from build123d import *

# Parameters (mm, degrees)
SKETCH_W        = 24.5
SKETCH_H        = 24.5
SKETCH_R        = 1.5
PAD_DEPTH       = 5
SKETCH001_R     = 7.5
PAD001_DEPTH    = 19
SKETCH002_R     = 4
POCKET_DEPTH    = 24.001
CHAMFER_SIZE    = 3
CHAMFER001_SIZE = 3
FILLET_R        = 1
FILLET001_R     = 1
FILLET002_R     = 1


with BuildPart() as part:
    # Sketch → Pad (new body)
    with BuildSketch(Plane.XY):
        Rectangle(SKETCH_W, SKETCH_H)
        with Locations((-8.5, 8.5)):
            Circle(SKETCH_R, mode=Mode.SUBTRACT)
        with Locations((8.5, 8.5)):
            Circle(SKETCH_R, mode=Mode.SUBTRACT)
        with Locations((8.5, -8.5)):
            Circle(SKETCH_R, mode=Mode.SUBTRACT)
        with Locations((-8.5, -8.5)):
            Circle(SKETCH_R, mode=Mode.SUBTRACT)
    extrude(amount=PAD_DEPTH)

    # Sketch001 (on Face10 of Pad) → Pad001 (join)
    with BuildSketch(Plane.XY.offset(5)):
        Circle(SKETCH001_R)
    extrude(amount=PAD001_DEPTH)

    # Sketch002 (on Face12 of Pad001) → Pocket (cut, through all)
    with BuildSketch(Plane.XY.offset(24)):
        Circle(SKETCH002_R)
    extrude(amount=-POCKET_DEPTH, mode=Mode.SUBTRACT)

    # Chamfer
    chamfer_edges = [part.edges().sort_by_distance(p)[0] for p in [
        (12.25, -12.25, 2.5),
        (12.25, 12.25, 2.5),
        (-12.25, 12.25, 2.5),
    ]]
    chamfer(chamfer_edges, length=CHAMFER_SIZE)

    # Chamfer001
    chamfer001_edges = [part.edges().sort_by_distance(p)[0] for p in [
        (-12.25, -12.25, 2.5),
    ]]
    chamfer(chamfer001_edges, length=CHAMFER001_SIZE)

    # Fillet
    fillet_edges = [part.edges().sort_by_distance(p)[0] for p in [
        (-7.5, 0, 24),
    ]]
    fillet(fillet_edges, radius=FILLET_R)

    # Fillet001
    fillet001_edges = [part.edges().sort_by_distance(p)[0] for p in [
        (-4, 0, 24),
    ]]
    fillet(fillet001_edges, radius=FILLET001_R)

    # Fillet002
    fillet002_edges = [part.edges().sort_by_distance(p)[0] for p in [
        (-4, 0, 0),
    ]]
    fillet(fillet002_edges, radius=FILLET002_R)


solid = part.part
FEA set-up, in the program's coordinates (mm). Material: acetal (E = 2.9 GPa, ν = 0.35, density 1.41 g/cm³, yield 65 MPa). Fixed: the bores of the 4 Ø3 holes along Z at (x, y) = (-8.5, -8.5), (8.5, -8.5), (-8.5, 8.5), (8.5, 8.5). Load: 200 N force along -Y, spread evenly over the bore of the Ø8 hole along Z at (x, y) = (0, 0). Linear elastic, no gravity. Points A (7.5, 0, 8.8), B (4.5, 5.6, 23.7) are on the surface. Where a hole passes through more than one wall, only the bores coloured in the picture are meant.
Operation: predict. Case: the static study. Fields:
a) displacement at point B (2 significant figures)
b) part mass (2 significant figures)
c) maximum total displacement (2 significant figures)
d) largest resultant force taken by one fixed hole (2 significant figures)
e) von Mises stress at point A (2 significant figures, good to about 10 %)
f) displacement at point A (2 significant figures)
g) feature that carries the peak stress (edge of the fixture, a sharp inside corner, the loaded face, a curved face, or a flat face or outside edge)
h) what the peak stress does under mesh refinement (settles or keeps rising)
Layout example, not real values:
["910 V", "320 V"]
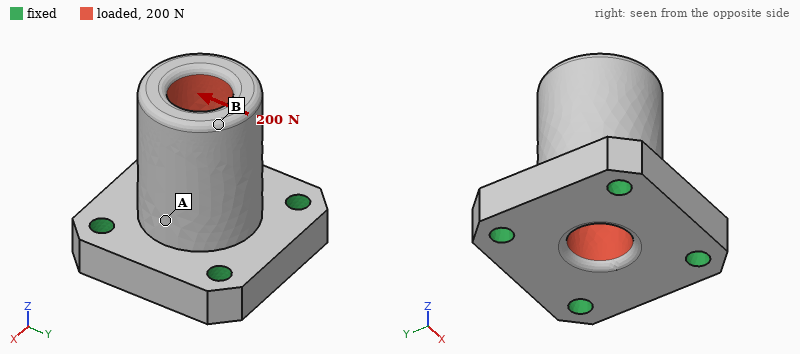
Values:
["75 µm", "6.9 g", "77 µm", "81 N", "2.1 MPa", "18 µm", "edge of the fixture", "keeps rising"]
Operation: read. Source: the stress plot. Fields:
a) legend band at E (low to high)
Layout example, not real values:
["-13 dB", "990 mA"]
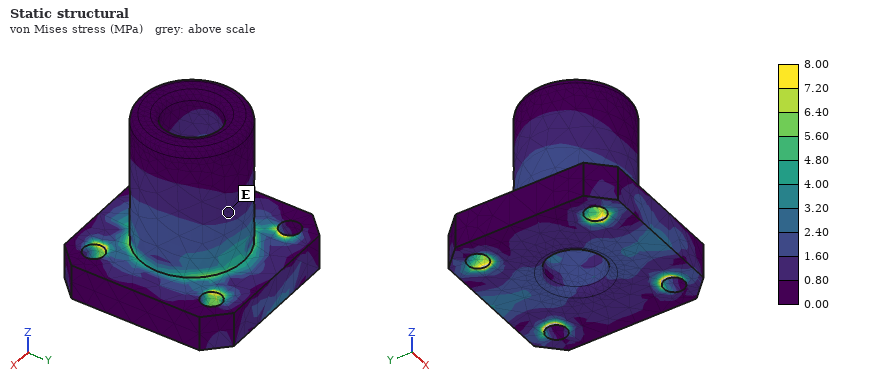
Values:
["0.80 to 1.60 MPa"]
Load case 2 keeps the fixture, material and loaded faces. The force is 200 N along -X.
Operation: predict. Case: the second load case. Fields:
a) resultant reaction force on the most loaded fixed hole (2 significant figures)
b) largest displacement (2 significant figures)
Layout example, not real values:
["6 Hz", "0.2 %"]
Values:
["81 N", "77 µm"]
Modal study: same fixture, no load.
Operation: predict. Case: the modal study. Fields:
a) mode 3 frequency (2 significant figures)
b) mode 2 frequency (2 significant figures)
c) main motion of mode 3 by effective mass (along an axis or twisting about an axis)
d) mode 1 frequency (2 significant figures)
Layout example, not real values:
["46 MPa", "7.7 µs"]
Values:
["9600 Hz", "4600 Hz", "along Z", "4600 Hz"]
